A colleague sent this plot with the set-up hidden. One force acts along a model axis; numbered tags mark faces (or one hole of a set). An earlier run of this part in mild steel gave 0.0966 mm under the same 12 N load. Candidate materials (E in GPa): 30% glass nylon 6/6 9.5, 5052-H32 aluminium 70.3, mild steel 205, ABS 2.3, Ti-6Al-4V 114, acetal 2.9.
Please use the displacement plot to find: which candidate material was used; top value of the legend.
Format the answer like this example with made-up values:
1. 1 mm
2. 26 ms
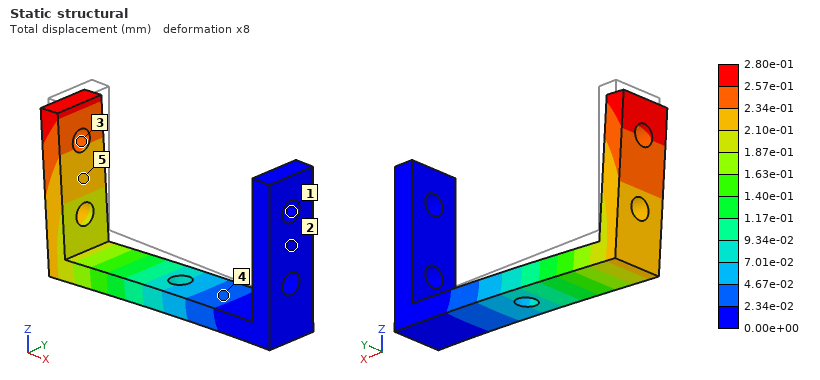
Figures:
1. 5052-H32 aluminium
2. 2.80e-01 mm
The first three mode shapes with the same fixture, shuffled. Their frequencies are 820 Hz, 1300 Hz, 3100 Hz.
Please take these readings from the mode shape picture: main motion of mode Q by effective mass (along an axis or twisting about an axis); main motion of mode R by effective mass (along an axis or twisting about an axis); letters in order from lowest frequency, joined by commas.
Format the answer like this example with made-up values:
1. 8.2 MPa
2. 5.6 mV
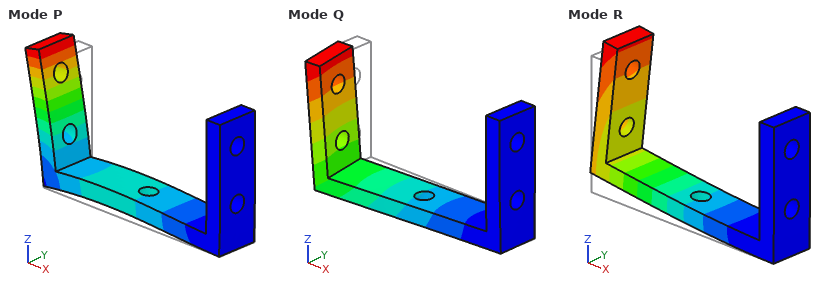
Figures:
1. along Y
2. along Z
3. R, Q, P
